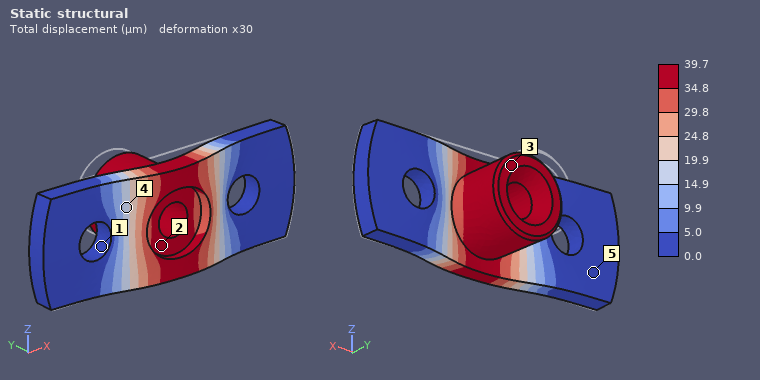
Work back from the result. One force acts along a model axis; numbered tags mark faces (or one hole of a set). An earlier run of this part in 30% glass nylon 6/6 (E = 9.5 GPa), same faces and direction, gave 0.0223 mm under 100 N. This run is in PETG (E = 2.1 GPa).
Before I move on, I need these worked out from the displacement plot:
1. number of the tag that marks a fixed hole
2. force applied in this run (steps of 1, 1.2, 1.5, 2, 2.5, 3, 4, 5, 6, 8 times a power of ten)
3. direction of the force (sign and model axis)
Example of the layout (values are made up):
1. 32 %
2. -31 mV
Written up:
1. 1
2. 40 N
3. -Y
